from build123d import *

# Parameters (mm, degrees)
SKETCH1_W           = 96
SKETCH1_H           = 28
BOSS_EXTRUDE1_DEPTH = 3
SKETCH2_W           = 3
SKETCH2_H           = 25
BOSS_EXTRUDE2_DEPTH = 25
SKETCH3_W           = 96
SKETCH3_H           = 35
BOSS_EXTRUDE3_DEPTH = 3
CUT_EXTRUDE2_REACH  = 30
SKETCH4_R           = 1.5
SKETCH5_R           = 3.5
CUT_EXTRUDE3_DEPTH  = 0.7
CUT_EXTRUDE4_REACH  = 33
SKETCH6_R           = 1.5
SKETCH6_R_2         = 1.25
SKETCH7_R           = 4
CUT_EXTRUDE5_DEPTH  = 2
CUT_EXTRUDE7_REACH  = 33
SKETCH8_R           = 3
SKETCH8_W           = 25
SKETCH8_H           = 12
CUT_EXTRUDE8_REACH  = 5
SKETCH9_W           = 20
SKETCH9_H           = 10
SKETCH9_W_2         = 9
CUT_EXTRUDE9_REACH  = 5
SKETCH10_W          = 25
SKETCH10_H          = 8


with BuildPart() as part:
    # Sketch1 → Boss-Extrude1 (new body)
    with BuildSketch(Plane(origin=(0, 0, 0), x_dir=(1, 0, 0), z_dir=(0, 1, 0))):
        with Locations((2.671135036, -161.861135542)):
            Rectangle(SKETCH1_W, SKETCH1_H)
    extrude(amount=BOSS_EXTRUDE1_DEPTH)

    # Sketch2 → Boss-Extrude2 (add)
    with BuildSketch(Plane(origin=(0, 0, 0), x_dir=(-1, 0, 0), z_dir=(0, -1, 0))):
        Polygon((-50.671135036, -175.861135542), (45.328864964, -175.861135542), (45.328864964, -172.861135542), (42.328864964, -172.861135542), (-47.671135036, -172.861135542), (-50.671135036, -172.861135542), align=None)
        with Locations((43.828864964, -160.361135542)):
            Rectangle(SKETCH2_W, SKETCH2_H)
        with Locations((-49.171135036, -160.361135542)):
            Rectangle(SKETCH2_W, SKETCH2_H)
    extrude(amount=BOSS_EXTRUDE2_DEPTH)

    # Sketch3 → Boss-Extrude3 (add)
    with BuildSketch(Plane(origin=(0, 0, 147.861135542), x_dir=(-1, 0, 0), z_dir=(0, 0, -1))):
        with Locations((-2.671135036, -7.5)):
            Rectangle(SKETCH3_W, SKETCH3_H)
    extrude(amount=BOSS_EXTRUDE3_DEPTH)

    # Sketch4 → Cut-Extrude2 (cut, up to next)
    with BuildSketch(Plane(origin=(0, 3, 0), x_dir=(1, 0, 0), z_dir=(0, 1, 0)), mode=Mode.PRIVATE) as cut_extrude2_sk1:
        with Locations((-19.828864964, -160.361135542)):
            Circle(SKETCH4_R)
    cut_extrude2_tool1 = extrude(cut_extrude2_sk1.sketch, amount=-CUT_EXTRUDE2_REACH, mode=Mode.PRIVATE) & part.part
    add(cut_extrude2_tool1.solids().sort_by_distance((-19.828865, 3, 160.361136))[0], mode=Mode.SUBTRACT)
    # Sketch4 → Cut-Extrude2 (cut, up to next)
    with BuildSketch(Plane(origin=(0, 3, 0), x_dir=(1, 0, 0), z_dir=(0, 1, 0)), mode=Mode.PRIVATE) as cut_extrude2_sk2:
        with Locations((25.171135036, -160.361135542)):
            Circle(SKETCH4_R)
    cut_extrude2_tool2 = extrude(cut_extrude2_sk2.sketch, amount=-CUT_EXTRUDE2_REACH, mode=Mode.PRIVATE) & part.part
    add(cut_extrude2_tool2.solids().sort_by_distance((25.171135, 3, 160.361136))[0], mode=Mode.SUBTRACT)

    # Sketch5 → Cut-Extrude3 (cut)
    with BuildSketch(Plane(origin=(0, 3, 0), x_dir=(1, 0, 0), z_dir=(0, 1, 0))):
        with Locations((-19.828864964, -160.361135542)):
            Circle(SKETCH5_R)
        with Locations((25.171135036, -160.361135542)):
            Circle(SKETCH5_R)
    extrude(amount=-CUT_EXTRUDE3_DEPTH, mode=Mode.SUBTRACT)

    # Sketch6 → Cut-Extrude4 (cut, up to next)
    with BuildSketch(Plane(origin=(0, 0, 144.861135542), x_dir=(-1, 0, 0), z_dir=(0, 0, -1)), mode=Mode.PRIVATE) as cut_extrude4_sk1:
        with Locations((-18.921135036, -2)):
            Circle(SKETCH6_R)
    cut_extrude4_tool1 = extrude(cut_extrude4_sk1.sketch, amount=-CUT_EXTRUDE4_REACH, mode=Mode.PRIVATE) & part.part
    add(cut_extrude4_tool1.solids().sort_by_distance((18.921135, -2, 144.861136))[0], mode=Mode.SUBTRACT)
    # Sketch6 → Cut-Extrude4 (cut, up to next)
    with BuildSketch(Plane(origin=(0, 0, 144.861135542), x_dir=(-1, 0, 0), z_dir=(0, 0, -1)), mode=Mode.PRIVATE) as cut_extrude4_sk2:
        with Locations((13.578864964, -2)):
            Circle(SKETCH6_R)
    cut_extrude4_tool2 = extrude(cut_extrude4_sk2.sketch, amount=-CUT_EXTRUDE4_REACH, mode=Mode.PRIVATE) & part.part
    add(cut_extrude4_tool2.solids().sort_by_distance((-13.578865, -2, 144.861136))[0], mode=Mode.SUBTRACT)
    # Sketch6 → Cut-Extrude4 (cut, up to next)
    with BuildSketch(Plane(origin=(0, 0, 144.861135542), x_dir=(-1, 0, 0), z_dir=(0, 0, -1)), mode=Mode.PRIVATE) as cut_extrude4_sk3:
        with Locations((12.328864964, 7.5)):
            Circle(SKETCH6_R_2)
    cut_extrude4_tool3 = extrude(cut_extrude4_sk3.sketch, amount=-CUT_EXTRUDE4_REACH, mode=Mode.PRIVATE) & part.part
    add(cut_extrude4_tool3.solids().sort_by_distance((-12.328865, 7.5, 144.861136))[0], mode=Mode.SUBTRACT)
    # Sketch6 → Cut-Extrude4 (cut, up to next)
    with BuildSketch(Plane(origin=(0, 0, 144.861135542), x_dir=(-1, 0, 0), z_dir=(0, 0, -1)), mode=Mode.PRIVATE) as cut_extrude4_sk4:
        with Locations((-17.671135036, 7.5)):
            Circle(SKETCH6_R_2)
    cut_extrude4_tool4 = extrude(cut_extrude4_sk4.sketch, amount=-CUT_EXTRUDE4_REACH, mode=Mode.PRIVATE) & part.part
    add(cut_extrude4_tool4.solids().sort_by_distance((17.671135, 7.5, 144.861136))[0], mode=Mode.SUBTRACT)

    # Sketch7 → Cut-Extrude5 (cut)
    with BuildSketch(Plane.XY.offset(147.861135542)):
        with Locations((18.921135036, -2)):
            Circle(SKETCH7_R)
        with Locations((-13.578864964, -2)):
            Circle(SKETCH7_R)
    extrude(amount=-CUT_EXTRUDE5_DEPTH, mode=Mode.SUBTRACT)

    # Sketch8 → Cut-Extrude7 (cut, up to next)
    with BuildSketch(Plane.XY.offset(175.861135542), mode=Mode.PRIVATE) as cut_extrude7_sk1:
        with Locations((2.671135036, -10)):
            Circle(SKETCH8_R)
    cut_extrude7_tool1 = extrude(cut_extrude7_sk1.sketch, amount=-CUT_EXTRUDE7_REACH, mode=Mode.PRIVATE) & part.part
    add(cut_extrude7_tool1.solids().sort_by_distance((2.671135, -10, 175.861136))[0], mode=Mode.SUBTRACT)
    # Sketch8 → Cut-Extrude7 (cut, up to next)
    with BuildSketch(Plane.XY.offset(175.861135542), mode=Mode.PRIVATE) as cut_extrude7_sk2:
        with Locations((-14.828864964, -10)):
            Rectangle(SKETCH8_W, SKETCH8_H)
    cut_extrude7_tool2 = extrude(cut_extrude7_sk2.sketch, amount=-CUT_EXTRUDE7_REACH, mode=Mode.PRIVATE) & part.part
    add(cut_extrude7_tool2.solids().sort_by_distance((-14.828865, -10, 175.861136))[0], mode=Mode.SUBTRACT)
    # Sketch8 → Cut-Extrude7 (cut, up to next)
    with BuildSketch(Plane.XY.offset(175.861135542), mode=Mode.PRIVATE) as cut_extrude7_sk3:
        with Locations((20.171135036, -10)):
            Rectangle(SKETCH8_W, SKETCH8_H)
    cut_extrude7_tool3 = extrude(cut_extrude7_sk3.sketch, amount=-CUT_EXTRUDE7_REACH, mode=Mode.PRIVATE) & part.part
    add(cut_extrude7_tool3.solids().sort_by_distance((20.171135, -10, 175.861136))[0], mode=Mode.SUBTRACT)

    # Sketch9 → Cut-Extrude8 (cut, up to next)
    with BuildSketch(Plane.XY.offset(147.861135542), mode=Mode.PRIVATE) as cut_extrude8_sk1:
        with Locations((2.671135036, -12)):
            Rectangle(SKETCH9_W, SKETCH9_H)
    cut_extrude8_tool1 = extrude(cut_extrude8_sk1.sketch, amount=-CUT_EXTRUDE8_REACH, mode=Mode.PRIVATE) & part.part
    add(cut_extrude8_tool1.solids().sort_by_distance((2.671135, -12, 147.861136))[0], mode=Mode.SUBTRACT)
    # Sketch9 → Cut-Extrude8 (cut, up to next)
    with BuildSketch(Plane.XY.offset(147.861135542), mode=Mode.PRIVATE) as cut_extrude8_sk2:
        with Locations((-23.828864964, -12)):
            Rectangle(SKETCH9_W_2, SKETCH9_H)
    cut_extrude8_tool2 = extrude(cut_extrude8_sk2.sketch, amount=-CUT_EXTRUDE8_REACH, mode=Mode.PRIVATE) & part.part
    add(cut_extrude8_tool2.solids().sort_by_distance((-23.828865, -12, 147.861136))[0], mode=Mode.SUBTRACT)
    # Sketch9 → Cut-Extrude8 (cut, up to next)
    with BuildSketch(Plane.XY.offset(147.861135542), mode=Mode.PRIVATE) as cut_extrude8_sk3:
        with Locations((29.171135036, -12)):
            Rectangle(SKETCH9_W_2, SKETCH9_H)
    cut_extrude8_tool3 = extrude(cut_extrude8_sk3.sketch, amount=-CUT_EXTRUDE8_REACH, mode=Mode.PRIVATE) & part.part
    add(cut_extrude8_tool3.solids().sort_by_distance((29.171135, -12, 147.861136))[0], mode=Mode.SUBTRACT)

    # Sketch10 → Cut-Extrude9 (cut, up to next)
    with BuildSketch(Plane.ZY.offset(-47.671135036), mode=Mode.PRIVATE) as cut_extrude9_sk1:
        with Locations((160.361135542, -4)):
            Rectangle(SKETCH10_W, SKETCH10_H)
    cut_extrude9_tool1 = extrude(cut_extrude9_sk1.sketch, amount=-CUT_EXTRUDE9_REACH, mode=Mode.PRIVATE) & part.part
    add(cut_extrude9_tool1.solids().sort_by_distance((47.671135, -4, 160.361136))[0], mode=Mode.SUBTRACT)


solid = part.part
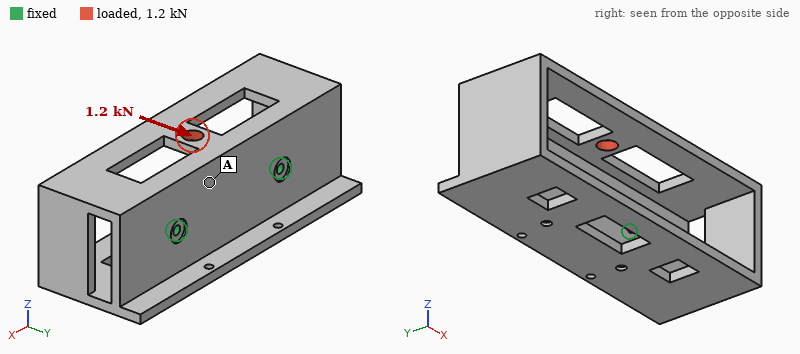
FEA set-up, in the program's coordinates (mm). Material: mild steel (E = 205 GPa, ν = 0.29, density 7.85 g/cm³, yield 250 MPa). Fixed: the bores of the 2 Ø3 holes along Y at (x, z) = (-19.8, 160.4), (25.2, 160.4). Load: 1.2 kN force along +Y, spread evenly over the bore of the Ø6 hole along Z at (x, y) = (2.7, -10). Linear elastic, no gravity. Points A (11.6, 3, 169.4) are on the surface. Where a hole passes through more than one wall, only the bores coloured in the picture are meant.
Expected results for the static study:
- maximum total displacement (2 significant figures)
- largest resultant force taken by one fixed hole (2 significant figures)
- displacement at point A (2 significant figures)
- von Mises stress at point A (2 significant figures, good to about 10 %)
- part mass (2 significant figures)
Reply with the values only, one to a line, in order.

0.17 mm
620 N
0.059 mm
47 MPa
200 g
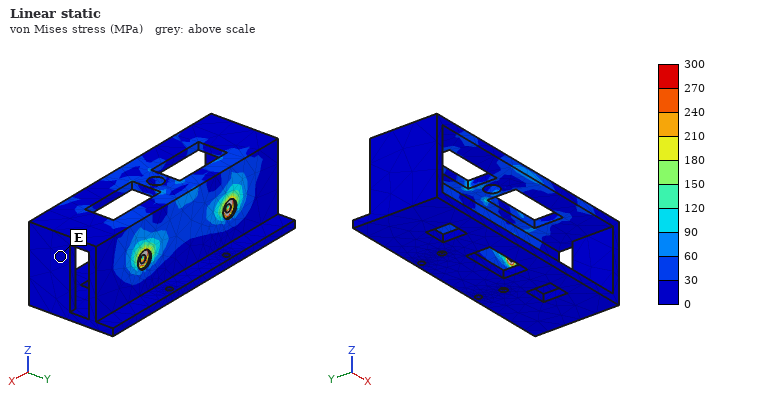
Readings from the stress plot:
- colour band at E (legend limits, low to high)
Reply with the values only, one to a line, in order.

0 to 30 MPa
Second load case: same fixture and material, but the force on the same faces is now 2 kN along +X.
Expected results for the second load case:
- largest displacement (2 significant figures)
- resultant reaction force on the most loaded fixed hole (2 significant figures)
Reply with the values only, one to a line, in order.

67 µm
1.3 kN
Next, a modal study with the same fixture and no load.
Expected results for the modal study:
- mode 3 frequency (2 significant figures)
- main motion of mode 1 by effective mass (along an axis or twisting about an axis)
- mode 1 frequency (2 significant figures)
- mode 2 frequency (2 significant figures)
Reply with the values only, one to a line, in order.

2400 Hz
along Z
1200 Hz
1900 Hz
